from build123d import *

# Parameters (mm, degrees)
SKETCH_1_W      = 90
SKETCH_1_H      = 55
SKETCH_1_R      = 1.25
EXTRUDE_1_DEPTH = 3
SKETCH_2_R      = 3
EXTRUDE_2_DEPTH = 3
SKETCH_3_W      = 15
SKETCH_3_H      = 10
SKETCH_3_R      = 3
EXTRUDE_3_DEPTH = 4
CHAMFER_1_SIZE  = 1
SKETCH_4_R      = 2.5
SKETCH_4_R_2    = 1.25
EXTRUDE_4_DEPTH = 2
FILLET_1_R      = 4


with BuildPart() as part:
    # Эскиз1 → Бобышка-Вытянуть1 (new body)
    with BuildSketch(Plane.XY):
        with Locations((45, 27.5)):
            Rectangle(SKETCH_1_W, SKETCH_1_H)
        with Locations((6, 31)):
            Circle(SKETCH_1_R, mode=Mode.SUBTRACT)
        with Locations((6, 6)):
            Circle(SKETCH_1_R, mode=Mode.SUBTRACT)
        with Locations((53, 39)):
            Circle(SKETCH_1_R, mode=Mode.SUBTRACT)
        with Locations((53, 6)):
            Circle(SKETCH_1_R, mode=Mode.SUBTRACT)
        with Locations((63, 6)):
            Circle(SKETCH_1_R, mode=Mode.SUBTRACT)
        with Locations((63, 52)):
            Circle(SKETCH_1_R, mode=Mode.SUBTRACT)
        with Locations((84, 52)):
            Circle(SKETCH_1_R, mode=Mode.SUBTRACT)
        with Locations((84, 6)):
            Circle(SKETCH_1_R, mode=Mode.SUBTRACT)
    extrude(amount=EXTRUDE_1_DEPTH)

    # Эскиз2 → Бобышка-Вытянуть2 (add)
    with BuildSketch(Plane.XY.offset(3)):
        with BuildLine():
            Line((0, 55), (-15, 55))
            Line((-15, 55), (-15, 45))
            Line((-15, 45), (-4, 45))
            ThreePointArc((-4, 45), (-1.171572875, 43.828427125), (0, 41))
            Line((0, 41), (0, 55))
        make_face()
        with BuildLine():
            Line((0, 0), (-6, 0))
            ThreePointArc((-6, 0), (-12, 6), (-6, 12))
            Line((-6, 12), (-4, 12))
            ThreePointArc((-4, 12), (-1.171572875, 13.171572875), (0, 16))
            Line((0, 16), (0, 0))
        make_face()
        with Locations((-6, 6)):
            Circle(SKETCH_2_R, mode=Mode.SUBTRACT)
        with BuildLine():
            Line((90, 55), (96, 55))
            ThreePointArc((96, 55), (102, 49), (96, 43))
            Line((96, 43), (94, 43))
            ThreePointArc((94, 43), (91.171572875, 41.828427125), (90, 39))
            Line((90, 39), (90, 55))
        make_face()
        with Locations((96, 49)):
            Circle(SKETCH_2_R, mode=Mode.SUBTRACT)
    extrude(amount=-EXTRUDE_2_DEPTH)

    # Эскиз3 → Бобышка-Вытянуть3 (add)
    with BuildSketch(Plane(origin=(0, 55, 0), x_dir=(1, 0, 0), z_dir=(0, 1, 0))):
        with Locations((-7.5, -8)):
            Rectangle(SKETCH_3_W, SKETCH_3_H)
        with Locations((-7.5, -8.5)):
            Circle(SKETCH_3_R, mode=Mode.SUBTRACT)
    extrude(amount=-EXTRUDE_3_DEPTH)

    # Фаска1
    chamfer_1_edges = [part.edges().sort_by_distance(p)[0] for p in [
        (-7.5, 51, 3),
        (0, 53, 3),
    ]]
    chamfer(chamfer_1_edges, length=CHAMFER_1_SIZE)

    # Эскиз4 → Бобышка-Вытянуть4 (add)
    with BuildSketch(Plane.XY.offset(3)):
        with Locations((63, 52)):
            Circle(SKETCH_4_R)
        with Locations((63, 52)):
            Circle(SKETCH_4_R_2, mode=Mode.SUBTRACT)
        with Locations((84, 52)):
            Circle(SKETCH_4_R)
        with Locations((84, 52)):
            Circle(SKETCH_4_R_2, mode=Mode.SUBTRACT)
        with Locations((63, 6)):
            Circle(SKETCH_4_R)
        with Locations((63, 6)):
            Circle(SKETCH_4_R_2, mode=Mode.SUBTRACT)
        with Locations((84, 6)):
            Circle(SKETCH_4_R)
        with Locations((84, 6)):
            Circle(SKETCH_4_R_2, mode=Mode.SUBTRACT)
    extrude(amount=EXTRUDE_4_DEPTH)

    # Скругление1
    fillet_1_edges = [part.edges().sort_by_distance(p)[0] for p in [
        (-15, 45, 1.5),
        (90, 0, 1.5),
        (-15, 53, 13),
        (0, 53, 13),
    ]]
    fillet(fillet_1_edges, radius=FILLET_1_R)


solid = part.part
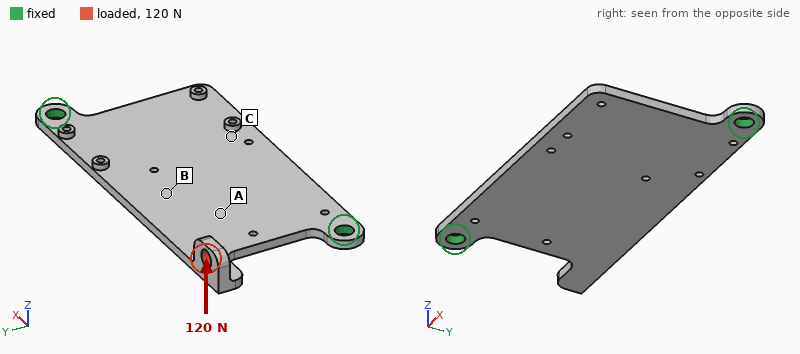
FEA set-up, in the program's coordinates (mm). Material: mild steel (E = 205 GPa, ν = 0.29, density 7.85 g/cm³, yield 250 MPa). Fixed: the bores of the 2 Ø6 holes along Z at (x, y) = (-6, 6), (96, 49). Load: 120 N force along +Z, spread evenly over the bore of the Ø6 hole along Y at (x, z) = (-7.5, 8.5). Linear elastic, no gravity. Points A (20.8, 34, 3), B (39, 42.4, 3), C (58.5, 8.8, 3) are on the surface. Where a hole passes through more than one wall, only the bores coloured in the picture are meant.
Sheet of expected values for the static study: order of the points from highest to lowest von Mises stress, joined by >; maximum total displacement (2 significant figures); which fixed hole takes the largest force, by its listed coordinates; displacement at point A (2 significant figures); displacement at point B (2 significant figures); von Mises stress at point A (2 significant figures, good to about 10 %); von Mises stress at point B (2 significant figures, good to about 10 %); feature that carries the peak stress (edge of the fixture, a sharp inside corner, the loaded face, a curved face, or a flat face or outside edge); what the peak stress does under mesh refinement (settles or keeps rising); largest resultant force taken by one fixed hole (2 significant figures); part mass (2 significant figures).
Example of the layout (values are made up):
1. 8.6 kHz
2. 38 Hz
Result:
1. A > B > C
2. 0.51 mm
3. (-6, 6)
4. 0.12 mm
5. 0.11 mm
6. 49 MPa
7. 34 MPa
8. edge of the fixture
9. keeps rising
10. 110 N
11. 130 g
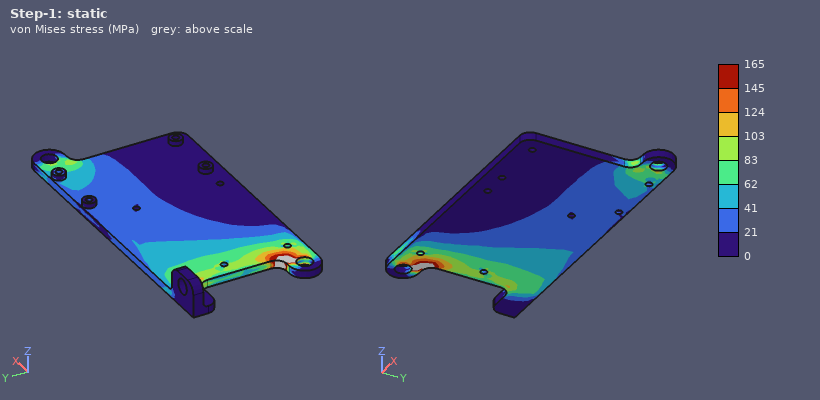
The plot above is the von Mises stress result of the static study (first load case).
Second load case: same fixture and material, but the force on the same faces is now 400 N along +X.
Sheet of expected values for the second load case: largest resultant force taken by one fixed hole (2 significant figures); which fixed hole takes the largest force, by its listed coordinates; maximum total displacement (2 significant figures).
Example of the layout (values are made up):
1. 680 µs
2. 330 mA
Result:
1. 260 N
2. (96, 49)
3. 0.25 mm
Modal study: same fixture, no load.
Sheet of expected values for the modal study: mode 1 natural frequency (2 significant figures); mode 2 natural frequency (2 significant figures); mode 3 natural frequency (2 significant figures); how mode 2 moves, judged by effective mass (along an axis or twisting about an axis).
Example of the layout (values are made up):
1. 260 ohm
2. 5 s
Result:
1. 680 Hz
2. 890 Hz
3. 1600 Hz
4. along Z
